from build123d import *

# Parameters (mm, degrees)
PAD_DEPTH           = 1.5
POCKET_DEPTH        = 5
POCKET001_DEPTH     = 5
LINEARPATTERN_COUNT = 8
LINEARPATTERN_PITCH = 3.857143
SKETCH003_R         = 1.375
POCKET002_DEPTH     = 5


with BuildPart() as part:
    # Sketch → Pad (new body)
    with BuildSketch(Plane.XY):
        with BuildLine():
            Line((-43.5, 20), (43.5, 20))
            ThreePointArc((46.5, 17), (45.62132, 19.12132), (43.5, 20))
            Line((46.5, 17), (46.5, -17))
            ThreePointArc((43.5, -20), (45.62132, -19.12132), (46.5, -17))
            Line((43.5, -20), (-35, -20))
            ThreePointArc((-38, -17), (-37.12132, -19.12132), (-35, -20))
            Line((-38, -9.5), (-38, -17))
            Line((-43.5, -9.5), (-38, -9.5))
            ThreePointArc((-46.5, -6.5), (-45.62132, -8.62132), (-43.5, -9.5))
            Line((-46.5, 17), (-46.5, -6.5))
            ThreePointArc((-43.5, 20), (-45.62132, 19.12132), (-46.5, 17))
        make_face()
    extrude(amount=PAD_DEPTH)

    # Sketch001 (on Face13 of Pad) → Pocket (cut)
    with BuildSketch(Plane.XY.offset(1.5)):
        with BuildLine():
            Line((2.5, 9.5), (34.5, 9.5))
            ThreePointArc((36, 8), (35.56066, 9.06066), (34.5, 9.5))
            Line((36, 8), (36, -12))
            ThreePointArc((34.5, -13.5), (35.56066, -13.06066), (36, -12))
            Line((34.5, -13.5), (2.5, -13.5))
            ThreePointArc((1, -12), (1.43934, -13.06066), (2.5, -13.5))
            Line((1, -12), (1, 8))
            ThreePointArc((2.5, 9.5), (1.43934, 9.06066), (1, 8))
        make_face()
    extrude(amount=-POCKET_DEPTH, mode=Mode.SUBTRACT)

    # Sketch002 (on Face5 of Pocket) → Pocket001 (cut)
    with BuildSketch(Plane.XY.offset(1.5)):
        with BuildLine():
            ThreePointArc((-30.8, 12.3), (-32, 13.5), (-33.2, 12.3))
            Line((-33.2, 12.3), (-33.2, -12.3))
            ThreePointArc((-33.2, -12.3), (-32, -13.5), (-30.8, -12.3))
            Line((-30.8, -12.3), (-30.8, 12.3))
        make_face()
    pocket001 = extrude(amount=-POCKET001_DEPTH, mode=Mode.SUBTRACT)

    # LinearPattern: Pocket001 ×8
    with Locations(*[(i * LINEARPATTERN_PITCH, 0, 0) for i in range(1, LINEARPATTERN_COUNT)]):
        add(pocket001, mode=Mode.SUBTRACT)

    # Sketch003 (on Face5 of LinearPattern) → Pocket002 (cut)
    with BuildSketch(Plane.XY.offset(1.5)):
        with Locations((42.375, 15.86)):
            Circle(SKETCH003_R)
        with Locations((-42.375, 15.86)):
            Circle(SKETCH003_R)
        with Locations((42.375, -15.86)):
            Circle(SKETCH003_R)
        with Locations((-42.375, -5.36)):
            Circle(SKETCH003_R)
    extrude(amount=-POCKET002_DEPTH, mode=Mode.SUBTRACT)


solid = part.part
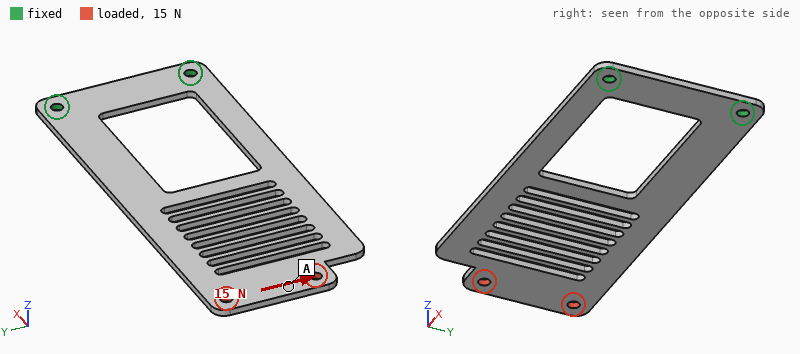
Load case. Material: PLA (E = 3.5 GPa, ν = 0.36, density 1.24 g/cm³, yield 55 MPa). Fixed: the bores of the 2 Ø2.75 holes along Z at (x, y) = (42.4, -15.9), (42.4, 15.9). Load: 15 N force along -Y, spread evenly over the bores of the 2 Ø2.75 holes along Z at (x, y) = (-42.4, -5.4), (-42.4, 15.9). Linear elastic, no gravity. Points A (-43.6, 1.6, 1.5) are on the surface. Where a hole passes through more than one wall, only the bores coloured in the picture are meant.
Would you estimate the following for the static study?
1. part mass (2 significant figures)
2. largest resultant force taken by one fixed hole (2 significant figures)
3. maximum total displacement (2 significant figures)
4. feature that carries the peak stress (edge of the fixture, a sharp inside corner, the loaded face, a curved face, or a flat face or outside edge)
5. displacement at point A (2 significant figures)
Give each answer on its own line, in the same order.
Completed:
4.3 g
37 N
0.96 mm
a curved face
0.94 mm
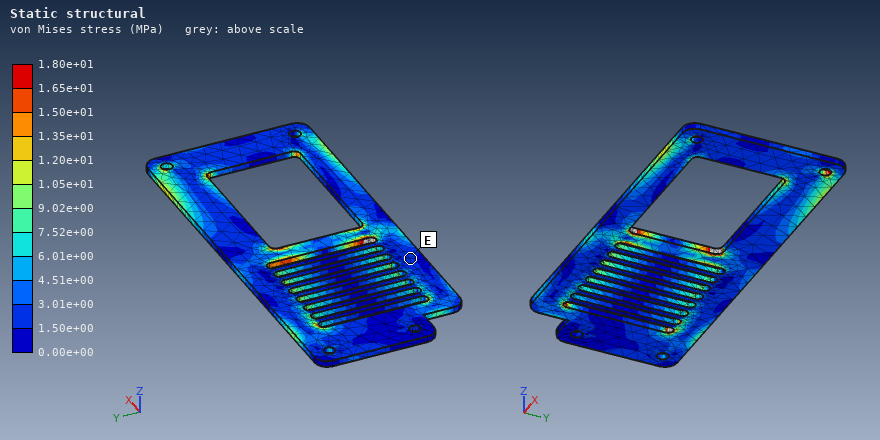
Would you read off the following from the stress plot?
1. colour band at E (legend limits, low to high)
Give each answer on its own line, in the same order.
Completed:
1.50e+00 to 3.01e+00 MPa
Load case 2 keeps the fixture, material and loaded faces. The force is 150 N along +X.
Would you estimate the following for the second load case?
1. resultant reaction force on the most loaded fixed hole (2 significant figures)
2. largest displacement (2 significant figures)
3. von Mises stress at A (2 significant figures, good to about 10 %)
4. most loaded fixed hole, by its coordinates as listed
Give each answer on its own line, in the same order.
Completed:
100 N
0.36 mm
2.5 MPa
(42.4, 15.9)
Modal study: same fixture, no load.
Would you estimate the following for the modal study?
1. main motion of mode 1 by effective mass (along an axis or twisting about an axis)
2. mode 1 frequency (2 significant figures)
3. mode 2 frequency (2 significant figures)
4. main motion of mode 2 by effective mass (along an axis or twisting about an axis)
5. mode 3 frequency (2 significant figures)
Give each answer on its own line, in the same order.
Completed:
along Z
42 Hz
190 Hz
twisting about X
270 Hz
